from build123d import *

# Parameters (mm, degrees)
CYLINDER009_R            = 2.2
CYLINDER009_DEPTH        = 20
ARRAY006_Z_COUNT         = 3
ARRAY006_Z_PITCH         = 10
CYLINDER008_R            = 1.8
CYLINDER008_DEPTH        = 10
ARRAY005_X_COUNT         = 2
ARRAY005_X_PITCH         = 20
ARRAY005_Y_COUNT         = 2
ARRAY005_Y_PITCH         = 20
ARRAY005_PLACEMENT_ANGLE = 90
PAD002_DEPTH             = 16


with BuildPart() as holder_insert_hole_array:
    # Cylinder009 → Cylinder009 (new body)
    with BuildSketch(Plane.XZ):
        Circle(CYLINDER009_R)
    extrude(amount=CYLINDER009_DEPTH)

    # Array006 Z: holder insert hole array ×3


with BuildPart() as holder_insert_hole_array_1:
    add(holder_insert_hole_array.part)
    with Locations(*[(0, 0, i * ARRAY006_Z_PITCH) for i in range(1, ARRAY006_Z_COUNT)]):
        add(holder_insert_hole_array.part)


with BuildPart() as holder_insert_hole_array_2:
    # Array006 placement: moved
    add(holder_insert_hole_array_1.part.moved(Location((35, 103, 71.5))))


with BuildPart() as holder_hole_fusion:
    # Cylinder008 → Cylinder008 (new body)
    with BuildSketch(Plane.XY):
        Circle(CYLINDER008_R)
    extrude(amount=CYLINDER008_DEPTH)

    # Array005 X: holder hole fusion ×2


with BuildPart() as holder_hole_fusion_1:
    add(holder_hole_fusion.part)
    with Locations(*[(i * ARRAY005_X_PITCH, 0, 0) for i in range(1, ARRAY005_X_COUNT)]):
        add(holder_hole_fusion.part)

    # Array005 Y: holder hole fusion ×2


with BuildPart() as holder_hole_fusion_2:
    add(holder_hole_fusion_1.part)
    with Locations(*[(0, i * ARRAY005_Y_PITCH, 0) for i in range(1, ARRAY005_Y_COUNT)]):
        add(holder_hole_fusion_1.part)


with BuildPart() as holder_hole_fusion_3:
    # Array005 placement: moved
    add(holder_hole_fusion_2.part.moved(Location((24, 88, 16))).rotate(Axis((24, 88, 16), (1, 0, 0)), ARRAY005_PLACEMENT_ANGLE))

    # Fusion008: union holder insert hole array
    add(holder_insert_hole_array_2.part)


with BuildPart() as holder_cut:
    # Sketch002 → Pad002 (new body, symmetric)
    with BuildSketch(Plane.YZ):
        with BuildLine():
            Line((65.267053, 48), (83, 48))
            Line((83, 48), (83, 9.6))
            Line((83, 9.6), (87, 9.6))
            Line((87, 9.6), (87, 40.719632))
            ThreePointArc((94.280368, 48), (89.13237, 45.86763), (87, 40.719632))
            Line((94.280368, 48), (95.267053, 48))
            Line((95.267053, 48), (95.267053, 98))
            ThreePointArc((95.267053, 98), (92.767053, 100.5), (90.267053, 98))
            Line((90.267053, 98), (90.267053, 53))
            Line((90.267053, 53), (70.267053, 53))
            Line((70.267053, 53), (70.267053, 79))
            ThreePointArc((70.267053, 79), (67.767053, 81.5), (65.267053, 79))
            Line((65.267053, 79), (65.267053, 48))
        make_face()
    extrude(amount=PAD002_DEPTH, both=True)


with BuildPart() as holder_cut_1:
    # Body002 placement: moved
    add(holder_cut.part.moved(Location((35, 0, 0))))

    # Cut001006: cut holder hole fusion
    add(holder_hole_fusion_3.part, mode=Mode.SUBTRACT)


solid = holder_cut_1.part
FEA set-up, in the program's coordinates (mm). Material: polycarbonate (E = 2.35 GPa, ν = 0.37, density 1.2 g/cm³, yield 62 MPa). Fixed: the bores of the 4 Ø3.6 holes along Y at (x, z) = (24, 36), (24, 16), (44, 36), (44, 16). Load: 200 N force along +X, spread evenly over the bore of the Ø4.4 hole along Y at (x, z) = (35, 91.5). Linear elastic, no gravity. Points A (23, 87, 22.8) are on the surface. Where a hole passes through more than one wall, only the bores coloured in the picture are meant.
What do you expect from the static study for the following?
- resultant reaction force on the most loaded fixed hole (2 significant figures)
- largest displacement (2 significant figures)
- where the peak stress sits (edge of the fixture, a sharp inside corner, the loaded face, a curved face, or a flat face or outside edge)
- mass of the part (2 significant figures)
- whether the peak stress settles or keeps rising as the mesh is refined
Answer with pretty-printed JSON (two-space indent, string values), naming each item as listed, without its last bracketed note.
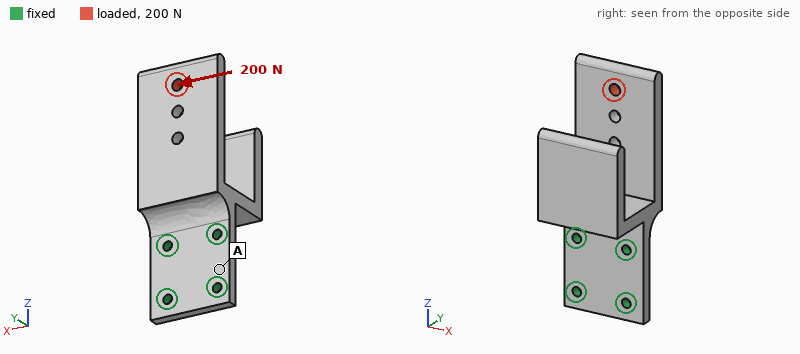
{
  "resultant reaction force on the most loaded fixed hole": "480 N",
  "largest displacement": "1.1 mm",
  "where the peak stress sits": "edge of the fixture",
  "mass of the part": "26 g",
  "whether the peak stress settles or keeps rising as the mesh is refined": "keeps rising"
}
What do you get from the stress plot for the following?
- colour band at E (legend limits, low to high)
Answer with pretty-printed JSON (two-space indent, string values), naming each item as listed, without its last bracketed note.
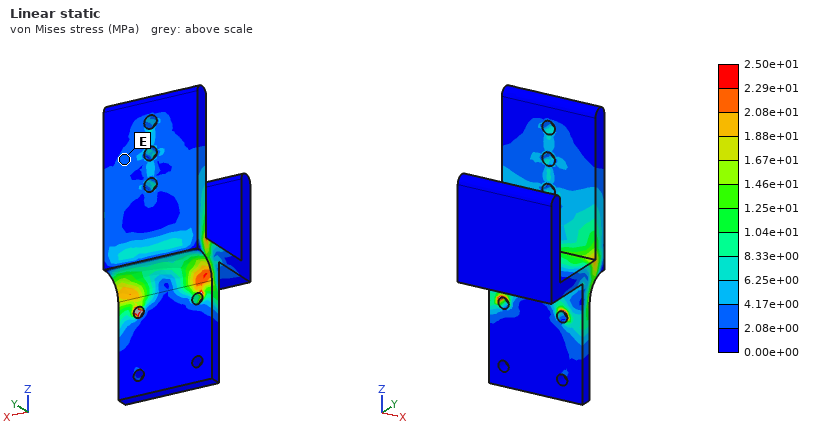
{
  "colour band at E": "2.08e+00 to 4.17e+00 MPa"
}
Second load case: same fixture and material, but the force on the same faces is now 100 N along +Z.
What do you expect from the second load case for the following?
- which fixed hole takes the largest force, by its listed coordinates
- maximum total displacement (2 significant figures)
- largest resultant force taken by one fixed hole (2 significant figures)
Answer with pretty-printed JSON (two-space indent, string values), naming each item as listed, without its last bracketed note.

{
  "which fixed hole takes the largest force, by its listed coordinates": "(44, 36)",
  "maximum total displacement": "1.0 mm",
  "largest resultant force taken by one fixed hole": "47 N"
}
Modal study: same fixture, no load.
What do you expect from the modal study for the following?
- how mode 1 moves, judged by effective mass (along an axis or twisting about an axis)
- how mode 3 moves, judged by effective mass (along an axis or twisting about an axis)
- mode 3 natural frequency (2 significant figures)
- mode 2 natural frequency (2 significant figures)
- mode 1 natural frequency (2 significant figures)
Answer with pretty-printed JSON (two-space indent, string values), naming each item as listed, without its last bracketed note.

{
  "how mode 1 moves, judged by effective mass": "along Y",
  "how mode 3 moves, judged by effective mass": "along X",
  "mode 3 natural frequency": "920 Hz",
  "mode 2 natural frequency": "560 Hz",
  "mode 1 natural frequency": "220 Hz"
}
